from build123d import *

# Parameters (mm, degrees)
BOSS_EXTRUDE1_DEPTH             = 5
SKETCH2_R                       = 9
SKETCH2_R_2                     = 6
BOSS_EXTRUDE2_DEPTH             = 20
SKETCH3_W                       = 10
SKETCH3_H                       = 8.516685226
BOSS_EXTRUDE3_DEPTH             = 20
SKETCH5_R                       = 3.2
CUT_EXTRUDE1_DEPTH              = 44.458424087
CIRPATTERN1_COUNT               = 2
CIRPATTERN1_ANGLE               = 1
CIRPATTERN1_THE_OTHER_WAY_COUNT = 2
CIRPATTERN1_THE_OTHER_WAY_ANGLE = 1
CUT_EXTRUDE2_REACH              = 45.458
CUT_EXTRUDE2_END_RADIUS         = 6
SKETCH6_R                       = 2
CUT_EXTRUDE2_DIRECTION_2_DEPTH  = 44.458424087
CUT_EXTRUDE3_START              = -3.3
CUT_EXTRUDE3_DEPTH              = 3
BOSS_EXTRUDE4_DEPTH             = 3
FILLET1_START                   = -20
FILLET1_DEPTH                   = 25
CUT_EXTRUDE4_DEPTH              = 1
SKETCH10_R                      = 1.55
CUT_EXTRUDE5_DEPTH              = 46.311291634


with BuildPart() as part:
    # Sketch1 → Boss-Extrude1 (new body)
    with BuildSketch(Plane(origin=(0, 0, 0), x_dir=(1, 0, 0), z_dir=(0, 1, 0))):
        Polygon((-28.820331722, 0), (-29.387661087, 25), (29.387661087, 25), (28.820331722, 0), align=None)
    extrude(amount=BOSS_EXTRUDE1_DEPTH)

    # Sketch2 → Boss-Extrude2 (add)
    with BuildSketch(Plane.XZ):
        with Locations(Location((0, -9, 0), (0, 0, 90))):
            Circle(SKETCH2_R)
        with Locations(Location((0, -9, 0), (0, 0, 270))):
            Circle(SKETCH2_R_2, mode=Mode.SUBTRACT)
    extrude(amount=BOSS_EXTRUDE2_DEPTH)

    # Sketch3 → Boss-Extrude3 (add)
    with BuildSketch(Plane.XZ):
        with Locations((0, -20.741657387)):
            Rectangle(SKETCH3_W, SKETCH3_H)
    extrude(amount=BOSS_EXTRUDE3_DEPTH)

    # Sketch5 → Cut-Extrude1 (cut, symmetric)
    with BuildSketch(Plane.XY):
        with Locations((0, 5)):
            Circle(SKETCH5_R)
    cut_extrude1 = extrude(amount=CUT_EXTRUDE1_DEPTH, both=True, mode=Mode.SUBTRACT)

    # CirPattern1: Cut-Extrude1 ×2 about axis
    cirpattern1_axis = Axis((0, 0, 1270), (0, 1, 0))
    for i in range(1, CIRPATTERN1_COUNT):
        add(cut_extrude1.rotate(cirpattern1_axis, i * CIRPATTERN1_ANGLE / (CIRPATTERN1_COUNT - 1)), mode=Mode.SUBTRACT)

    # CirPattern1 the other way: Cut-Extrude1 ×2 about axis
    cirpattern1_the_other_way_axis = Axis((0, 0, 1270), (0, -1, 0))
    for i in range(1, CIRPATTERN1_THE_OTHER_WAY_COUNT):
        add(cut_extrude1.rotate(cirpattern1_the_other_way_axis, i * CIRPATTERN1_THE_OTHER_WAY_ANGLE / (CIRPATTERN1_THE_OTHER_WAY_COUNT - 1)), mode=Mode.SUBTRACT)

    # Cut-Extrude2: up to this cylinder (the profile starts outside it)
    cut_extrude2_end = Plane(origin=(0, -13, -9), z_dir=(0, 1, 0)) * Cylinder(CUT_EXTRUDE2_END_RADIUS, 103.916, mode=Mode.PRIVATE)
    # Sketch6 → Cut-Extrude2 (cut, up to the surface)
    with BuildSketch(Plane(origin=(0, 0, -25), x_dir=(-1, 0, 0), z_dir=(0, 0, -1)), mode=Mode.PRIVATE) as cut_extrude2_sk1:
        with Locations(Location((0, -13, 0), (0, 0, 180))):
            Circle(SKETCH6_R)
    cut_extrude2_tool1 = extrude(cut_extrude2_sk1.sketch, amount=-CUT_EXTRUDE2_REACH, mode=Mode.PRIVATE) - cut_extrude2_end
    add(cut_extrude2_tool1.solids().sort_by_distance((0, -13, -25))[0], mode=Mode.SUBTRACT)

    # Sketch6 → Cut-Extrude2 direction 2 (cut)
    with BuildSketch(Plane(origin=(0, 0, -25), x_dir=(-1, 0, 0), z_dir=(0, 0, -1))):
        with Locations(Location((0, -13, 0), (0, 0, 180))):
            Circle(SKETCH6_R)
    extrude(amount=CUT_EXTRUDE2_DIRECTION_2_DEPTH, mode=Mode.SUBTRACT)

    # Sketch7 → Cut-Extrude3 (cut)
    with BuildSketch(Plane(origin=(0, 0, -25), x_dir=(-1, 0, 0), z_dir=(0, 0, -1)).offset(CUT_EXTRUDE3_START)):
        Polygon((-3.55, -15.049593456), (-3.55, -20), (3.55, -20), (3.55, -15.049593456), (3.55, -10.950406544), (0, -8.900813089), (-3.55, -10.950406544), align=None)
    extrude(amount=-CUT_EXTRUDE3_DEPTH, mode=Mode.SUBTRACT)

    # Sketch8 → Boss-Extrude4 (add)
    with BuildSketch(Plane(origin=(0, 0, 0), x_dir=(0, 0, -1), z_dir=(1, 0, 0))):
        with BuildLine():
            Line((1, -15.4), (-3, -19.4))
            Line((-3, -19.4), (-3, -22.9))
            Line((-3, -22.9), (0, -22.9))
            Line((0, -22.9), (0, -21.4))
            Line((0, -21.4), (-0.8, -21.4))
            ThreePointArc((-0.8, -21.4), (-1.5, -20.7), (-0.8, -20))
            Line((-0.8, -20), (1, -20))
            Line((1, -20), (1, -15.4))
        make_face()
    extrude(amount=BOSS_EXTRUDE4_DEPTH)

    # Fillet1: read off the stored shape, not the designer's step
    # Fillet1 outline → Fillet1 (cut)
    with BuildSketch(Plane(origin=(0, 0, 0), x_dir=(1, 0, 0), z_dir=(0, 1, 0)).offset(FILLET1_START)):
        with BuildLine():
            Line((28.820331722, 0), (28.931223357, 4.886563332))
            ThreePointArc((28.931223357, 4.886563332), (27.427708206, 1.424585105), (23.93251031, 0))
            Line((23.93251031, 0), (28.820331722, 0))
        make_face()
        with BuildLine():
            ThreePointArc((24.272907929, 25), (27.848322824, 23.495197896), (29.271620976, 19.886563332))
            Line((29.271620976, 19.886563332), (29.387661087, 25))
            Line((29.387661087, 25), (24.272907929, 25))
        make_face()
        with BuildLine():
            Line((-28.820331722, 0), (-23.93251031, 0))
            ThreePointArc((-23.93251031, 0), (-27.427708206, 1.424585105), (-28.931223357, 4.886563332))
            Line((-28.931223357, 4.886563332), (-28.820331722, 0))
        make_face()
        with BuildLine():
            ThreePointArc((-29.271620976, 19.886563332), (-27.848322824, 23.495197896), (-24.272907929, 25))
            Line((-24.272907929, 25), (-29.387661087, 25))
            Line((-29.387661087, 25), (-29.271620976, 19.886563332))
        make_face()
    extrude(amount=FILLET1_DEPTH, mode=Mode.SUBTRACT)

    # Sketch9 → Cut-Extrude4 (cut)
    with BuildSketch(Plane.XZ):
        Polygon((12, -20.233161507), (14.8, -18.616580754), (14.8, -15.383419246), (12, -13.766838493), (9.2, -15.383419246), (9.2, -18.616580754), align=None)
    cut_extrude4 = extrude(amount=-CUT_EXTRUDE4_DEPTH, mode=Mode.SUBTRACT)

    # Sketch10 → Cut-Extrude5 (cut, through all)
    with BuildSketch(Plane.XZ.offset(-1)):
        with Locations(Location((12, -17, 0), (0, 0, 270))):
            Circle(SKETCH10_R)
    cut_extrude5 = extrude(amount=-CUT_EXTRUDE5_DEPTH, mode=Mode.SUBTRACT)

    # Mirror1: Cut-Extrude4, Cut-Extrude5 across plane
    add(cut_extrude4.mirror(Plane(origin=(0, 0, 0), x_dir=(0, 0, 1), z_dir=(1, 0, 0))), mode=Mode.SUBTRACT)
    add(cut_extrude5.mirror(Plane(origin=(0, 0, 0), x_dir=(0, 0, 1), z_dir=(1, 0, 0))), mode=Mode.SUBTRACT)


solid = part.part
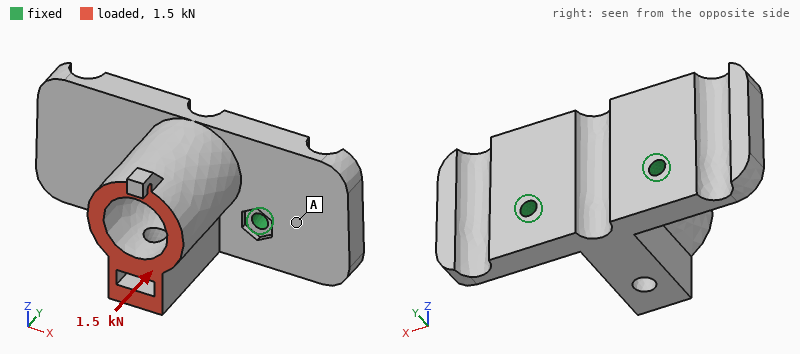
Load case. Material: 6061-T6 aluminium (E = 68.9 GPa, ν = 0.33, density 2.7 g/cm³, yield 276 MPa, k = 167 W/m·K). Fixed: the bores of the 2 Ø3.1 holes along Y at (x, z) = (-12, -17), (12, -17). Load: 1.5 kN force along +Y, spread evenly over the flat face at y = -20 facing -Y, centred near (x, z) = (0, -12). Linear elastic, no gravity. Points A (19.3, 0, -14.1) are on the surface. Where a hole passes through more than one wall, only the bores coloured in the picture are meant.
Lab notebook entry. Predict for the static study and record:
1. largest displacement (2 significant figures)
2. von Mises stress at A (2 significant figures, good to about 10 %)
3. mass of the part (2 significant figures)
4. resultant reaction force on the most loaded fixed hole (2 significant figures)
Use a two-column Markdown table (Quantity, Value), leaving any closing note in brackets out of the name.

| Quantity | Value |
|---|---|
| largest displacement | 60 µm |
| von Mises stress at A | 13 MPa |
| mass of the part | 27 g |
| resultant reaction force on the most loaded fixed hole | 850 N |
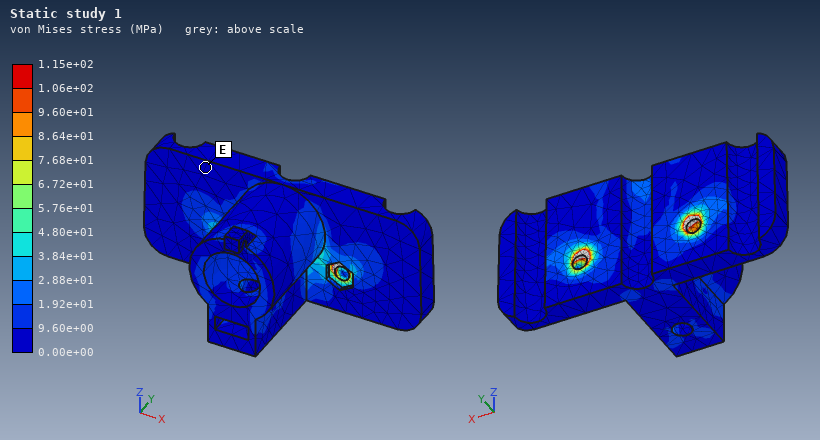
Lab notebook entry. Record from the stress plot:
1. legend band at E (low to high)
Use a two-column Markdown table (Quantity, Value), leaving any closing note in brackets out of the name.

| Quantity | Value |
|---|---|
| legend band at E | 0.00e+00 to 9.60e+00 MPa |
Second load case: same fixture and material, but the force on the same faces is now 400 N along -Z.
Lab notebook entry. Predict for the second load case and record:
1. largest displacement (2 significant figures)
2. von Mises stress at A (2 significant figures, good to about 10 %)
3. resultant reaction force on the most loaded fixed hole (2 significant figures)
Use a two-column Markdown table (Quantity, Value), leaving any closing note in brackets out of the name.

| Quantity | Value |
|---|---|
| largest displacement | 87 µm |
| von Mises stress at A | 15 MPa |
| resultant reaction force on the most loaded fixed hole | 280 N |
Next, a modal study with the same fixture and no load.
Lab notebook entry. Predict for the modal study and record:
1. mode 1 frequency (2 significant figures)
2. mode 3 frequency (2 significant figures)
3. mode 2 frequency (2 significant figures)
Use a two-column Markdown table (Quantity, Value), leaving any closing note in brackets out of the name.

| Quantity | Value |
|---|---|
| mode 1 frequency | 5000 Hz |
| mode 3 frequency | 8800 Hz |
| mode 2 frequency | 8700 Hz |
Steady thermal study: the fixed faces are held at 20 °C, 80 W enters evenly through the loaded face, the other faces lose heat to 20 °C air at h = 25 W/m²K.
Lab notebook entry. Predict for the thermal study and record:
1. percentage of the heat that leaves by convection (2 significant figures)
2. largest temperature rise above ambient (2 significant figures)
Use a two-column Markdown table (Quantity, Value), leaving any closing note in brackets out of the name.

| Quantity | Value |
|---|---|
| percentage of the heat that leaves by convection | 5.4 % |
| largest temperature rise above ambient | 74 K |
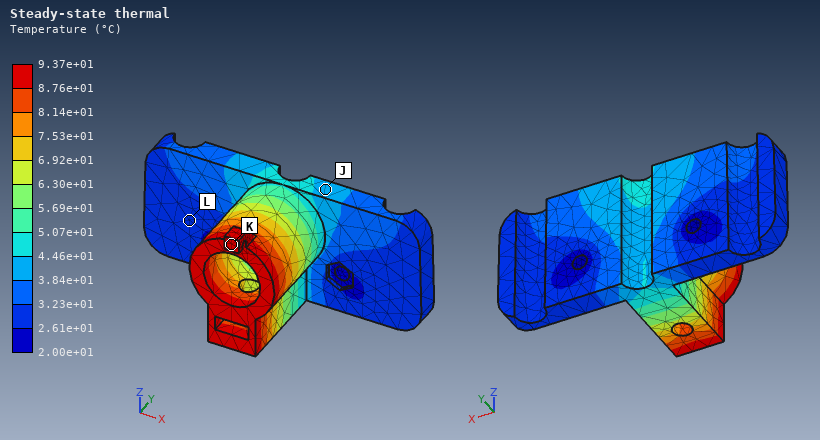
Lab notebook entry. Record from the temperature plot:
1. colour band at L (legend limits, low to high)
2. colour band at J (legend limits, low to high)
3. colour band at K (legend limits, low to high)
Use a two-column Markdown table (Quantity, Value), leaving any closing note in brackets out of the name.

| Quantity | Value |
|---|---|
| colour band at L | 2.61e+01 to 3.23e+01 °C |
| colour band at J | 3.84e+01 to 4.46e+01 °C |
| colour band at K | 8.76e+01 to 9.37e+01 °C |
